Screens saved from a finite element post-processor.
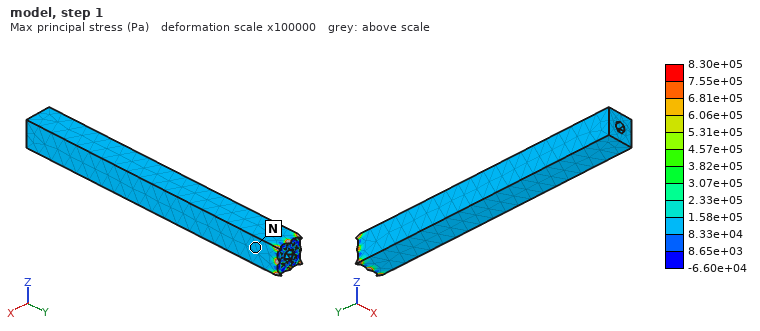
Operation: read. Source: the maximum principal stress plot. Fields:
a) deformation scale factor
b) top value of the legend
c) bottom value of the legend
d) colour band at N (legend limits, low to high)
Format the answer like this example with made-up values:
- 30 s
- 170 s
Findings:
- 100000
- 8.30e+05 Pa
- -6.60e+04 Pa
- 8.33e+04 to 1.58e+05 Pa
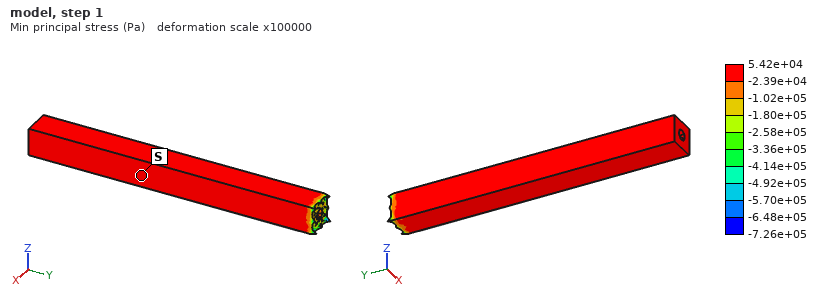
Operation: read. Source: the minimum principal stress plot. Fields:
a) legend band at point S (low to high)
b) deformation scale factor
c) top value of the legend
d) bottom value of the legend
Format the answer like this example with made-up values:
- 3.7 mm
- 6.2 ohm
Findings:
- -2.39e+04 to 5.42e+04 Pa
- 100000
- 5.42e+04 Pa
- -7.26e+05 Pa
